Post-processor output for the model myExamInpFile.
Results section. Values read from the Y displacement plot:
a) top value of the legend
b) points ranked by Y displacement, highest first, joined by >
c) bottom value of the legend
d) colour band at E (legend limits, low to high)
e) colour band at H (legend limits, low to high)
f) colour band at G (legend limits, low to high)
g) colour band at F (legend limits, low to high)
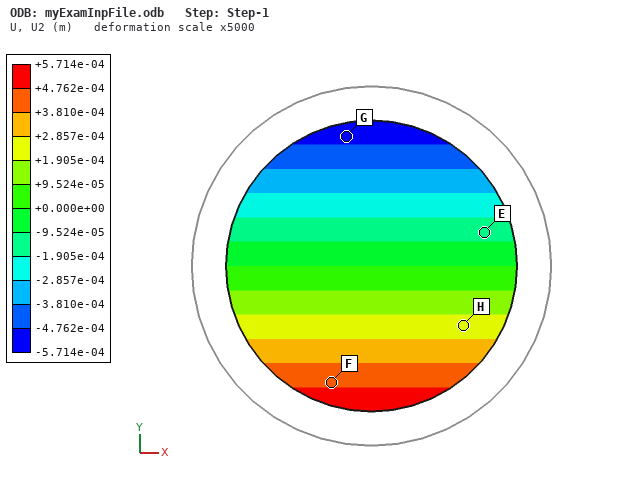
+5.714e-04 m
F > H > E > G
-5.714e-04 m
-1.905e-04 to -9.524e-05 m
+1.905e-04 to +2.857e-04 m
-5.714e-04 to -4.762e-04 m
+3.810e-04 to +4.762e-04 m
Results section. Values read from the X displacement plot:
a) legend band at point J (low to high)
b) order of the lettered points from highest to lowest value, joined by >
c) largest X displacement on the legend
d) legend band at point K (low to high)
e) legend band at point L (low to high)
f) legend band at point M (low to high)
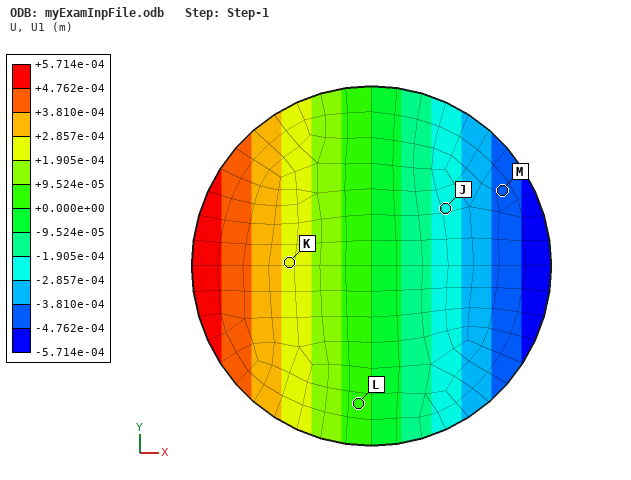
-2.857e-04 to -1.905e-04 m
K > L > J > M
+5.714e-04 m
+1.905e-04 to +2.857e-04 m
+0.000e+00 to +9.524e-05 m
-4.762e-04 to -3.810e-04 m
